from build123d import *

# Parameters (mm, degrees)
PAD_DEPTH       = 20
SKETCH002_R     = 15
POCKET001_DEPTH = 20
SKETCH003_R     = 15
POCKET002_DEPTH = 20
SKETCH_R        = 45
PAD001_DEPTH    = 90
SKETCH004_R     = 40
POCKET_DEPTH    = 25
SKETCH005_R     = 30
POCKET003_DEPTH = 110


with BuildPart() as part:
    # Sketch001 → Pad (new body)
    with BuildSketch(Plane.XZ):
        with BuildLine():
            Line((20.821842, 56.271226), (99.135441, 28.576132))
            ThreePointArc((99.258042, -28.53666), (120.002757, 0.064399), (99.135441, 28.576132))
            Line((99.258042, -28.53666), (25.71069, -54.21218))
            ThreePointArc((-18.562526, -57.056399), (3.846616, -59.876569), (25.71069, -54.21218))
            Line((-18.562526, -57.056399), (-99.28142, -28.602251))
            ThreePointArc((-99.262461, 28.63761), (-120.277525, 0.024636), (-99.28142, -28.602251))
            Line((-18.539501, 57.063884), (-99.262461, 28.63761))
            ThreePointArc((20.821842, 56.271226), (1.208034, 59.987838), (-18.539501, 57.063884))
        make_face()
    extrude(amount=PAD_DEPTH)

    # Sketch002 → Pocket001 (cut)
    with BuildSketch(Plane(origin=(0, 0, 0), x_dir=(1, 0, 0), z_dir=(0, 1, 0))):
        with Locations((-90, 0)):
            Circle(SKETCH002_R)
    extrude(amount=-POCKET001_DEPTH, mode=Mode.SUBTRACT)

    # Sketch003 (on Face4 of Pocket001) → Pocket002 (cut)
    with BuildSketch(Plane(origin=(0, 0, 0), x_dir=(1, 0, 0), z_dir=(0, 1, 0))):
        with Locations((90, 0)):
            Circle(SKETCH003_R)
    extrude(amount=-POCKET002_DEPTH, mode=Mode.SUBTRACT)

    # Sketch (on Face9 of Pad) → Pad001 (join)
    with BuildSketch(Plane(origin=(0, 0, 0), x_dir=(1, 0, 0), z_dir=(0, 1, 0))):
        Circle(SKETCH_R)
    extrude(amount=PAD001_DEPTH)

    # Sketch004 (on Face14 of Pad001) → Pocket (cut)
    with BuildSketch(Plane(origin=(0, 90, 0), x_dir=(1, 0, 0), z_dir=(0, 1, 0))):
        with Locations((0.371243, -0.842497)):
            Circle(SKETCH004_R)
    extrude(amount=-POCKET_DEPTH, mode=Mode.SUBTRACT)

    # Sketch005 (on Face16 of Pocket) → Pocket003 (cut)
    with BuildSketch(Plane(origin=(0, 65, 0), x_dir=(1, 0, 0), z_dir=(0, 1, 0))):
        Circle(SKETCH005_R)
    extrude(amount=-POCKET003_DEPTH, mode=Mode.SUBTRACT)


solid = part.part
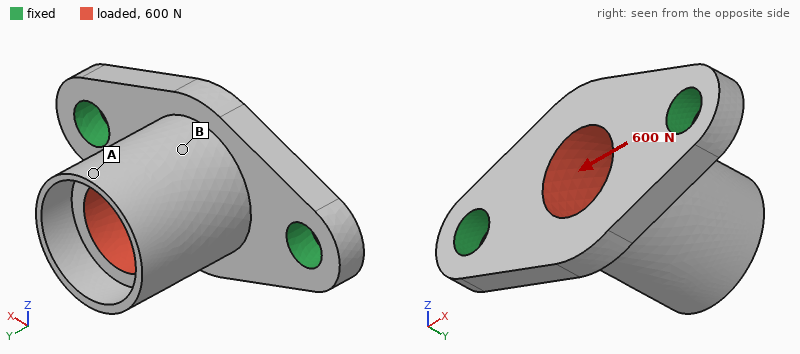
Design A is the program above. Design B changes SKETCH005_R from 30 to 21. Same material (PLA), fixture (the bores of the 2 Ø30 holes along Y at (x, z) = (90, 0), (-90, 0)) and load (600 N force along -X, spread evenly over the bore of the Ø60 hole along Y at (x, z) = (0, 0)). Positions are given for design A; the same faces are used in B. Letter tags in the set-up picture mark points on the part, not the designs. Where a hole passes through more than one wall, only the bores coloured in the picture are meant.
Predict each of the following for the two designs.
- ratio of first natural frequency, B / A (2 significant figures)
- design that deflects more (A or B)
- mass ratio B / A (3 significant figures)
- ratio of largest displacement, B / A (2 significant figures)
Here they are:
0.93
A
1.21
0.86
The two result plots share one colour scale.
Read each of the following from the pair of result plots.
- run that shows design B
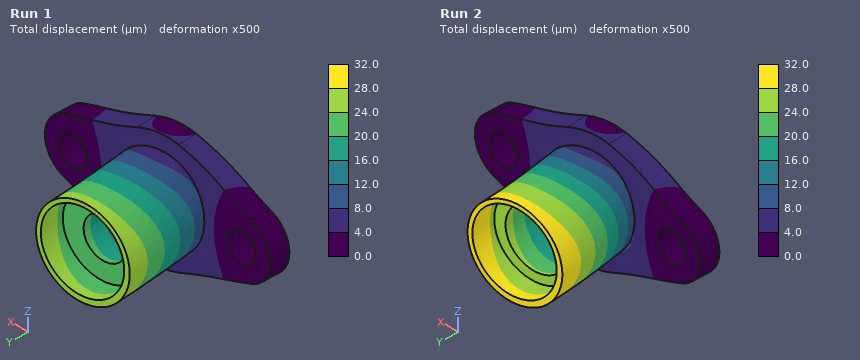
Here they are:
Run 1
